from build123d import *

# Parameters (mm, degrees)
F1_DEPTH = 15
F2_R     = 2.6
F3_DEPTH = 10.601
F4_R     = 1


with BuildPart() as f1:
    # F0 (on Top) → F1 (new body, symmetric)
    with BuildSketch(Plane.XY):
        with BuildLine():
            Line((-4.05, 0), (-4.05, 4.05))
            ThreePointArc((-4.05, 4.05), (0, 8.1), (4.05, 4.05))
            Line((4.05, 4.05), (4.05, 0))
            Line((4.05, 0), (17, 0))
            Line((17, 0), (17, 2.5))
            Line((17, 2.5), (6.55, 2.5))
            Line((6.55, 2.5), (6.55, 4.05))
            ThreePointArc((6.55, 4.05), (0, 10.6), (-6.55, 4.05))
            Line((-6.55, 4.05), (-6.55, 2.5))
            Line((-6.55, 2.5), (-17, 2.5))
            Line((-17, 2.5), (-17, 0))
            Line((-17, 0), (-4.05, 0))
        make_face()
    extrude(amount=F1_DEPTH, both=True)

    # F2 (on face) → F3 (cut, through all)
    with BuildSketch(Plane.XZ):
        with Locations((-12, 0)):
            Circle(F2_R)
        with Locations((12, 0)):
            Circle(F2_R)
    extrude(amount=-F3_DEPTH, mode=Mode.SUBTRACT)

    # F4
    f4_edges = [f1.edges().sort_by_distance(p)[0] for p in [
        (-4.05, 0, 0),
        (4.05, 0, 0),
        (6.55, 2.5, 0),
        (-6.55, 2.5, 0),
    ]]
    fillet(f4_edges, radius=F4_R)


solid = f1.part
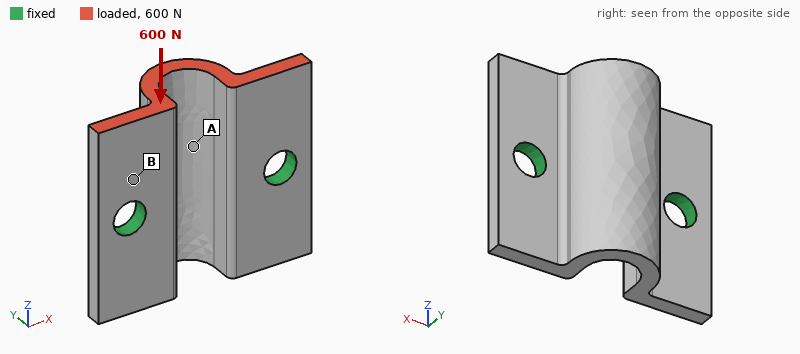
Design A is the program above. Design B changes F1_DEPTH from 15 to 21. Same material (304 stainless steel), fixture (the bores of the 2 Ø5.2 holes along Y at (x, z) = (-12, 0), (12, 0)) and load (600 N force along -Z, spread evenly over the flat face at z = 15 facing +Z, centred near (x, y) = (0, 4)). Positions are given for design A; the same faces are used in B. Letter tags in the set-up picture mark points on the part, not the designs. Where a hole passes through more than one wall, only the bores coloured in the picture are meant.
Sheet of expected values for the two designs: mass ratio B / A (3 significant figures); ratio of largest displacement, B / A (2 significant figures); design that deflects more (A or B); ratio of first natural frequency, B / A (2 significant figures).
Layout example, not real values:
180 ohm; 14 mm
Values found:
1.41; 1.2; B; 0.62
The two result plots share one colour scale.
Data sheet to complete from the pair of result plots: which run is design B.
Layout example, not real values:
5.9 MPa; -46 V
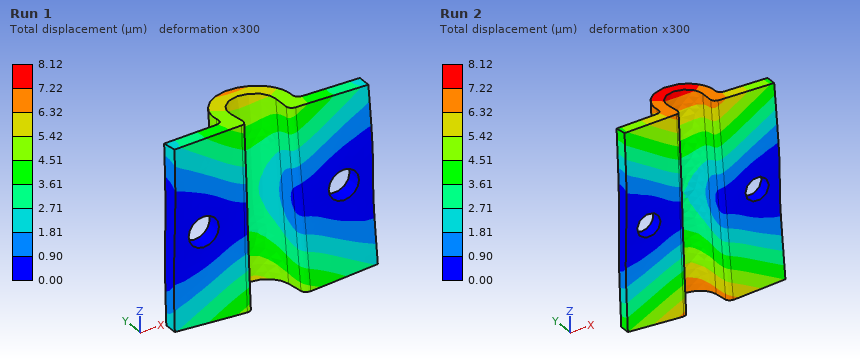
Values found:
Run 2
